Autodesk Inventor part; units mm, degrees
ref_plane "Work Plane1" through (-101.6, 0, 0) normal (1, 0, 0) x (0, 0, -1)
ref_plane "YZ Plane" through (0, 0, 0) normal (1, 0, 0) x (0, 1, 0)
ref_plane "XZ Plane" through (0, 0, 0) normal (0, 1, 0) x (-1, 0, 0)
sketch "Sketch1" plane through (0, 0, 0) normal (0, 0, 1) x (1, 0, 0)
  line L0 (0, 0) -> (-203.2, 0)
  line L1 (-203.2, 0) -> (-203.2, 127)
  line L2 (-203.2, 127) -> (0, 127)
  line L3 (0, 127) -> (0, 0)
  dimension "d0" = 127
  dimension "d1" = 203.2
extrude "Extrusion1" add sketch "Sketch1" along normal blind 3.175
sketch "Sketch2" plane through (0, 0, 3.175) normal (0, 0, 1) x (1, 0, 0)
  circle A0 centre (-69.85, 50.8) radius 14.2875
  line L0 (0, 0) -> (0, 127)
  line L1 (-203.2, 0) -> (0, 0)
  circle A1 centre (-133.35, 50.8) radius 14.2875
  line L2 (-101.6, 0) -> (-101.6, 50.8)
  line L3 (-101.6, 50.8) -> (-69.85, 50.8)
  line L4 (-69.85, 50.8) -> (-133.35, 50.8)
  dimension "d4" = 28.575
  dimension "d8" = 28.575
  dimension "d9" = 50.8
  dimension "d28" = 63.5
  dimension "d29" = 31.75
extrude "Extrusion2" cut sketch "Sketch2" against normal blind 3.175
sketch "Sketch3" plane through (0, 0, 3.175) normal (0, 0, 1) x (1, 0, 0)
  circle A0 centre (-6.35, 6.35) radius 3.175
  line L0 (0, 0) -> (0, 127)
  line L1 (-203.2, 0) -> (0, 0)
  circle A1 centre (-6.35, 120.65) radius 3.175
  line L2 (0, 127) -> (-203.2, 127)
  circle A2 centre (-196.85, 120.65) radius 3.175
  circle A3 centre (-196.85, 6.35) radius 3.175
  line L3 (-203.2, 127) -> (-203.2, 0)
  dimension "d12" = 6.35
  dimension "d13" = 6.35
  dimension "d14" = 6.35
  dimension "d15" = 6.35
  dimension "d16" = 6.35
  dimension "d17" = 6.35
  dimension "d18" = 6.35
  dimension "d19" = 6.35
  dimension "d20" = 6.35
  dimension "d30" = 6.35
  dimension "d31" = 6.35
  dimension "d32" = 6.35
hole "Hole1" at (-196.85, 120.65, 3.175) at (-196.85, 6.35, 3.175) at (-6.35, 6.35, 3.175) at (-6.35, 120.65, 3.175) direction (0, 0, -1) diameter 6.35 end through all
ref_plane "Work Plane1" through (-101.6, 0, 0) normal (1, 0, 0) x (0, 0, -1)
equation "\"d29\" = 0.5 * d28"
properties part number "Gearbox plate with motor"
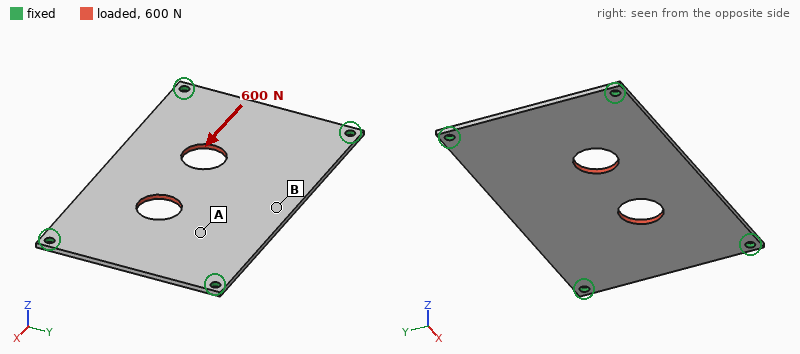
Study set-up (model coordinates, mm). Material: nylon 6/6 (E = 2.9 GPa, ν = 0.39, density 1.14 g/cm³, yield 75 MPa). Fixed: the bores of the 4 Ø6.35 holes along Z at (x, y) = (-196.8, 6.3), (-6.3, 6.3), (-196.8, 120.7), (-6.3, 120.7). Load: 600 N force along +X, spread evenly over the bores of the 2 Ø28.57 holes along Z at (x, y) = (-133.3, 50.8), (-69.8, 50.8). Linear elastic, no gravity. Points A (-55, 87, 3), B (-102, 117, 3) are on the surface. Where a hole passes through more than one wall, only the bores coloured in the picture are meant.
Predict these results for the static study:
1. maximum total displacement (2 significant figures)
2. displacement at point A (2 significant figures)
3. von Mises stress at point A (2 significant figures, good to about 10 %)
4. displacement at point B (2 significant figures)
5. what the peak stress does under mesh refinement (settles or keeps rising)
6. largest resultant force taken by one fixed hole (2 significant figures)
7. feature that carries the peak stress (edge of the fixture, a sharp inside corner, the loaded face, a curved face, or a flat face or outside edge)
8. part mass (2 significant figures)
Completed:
57 µm
34 µm
0.90 MPa
27 µm
keeps rising
170 N
edge of the fixture
88 g
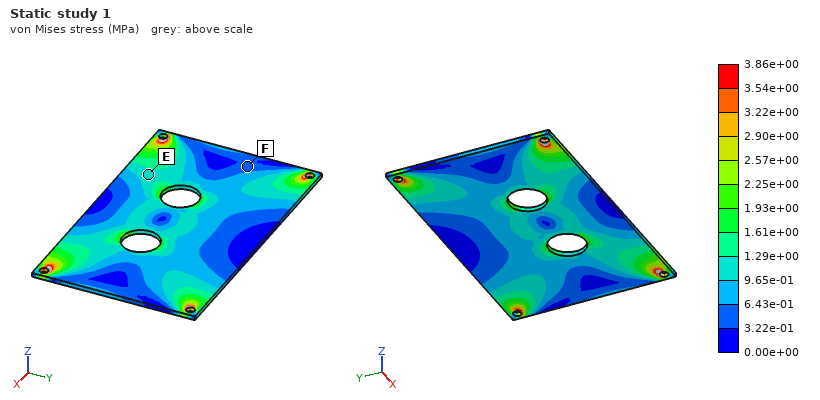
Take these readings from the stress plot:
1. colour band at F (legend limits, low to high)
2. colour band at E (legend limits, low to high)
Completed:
3.22e-01 to 6.43e-01 MPa
9.65e-01 to 1.29e+00 MPa
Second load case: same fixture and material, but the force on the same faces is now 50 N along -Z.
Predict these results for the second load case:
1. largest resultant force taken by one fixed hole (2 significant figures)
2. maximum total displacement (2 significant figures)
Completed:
16 N
2.6 mm
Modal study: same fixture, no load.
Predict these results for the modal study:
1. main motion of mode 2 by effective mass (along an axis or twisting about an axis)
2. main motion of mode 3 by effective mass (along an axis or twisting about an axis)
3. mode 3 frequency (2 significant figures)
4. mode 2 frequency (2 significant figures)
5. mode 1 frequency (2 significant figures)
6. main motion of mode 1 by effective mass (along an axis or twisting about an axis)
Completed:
twisting about X
twisting about Y
310 Hz
200 Hz
120 Hz
along Z
